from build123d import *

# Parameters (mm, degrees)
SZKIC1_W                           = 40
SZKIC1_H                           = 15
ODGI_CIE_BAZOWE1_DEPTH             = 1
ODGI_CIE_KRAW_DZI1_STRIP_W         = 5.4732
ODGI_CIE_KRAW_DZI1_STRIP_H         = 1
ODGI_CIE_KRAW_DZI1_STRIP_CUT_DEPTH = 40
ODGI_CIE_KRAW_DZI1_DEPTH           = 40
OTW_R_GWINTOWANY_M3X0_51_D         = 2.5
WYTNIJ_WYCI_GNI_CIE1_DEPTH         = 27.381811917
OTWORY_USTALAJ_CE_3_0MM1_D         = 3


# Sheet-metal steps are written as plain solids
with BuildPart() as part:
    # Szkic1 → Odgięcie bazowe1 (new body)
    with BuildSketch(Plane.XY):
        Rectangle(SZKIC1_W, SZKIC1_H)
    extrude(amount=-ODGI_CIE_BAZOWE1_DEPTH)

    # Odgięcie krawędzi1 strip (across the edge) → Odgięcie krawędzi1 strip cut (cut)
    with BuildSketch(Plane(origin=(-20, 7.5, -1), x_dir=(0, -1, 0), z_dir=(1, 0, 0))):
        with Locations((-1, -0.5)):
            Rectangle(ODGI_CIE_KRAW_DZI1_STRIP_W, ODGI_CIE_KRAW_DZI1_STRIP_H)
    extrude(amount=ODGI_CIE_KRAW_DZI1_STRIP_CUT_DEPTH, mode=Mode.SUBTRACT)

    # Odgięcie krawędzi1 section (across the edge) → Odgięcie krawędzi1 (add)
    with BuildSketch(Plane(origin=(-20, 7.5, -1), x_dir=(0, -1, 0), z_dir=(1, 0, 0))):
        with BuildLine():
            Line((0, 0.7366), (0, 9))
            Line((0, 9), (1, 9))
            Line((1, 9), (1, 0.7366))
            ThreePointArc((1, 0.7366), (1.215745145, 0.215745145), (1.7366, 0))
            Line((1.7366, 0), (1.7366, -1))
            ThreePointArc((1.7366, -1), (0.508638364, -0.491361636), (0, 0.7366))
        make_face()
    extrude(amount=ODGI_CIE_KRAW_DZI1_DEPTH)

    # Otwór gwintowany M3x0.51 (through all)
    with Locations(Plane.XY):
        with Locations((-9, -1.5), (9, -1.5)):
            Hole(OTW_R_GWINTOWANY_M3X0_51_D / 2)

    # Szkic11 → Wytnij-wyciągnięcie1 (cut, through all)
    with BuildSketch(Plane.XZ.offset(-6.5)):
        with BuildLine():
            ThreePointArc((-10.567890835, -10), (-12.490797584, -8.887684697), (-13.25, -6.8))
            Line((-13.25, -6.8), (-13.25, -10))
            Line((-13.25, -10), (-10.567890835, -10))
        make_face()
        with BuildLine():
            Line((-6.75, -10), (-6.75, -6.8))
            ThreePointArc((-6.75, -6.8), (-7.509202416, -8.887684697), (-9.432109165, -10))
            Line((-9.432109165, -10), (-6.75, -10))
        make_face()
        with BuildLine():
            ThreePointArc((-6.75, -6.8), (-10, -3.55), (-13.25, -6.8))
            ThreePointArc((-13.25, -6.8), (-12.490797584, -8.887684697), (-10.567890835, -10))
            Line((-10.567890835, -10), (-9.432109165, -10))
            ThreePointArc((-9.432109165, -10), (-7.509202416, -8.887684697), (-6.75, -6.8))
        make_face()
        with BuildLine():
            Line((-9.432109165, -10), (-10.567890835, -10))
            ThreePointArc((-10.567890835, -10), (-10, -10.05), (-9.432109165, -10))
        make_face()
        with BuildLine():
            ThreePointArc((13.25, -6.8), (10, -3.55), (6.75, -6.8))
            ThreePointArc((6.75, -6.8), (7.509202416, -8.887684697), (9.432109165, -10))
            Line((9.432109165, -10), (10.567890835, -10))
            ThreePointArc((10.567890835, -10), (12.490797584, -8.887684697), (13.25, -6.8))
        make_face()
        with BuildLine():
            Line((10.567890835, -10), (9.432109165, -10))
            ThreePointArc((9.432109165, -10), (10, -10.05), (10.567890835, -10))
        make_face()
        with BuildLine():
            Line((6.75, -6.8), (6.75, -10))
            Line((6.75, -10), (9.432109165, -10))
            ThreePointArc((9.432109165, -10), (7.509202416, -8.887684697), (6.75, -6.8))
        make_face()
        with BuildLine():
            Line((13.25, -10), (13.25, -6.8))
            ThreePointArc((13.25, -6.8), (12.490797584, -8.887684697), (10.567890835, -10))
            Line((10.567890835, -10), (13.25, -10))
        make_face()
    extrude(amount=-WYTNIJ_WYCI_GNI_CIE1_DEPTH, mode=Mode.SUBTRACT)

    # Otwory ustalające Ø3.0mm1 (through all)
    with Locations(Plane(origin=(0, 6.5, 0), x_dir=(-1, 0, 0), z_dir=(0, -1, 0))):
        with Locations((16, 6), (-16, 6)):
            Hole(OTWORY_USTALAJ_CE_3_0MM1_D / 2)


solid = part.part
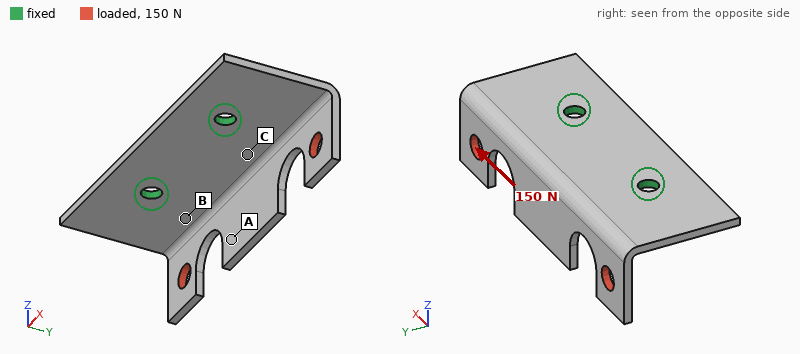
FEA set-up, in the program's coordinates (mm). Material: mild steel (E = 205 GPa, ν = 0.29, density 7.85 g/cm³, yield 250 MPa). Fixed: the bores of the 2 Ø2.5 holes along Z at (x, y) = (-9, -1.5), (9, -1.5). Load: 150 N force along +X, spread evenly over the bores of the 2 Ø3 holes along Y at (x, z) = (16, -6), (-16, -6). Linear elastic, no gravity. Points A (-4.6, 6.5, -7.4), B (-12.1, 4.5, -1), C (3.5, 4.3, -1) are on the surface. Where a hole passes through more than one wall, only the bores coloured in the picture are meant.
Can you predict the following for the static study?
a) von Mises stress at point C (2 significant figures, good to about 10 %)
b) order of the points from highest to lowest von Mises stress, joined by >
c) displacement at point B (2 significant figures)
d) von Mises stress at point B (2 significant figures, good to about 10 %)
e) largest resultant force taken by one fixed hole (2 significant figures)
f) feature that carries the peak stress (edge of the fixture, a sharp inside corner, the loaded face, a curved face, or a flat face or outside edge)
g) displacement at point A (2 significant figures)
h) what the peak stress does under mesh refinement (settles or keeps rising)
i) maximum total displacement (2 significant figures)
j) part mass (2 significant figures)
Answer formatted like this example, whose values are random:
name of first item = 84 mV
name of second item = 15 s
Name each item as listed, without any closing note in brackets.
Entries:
von Mises stress at point C = 52 MPa
order of the points from highest to lowest von Mises stress, joined by > = C > B > A
displacement at point B = 15 µm
von Mises stress at point B = 25 MPa
largest resultant force taken by one fixed hole = 110 N
feature that carries the peak stress = edge of the fixture
displacement at point A = 15 µm
what the peak stress does under mesh refinement = keeps rising
maximum total displacement = 65 µm
part mass = 6.6 g
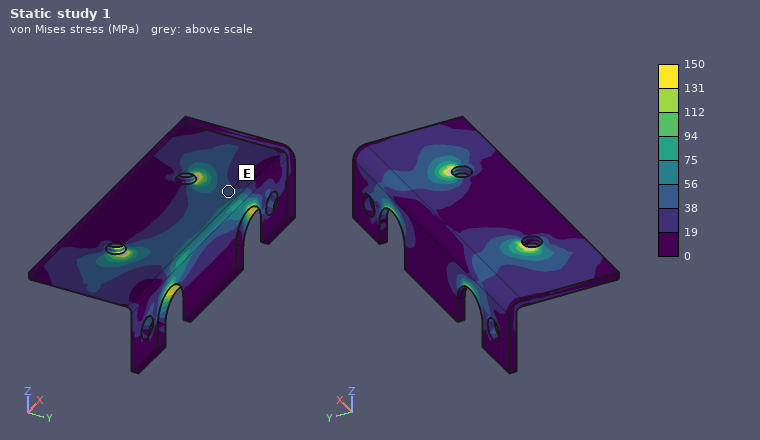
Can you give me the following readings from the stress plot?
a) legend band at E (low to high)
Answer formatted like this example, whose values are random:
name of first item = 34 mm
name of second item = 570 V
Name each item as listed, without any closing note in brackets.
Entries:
legend band at E = 38 to 56 MPa
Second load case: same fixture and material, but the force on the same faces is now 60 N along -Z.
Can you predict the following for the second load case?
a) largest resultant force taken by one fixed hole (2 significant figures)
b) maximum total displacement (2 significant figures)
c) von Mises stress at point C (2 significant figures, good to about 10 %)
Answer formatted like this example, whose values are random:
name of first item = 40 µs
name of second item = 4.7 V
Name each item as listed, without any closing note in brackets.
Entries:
largest resultant force taken by one fixed hole = 33 N
maximum total displacement = 46 µm
von Mises stress at point C = 29 MPa
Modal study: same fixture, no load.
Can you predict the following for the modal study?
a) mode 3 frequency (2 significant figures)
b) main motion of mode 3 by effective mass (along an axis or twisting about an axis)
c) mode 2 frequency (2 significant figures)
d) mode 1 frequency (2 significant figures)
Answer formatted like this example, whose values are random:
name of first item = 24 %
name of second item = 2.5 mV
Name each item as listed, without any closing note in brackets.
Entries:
mode 3 frequency = 7600 Hz
main motion of mode 3 by effective mass = twisting about Y
mode 2 frequency = 4300 Hz
mode 1 frequency = 3900 Hz
